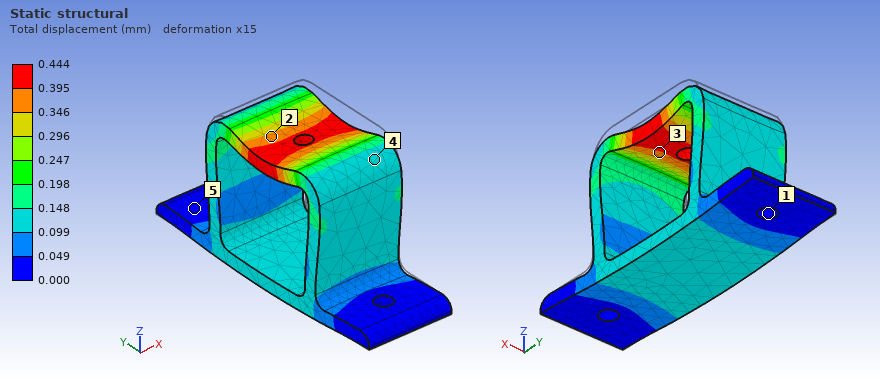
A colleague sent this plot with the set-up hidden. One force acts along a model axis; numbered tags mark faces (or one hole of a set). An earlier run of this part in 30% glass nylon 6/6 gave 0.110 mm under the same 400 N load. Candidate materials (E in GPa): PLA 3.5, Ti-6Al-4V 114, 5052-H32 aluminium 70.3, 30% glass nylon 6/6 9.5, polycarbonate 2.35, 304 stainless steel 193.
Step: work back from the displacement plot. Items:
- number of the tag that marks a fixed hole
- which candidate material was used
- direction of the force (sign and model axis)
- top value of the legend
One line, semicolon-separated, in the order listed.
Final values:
1; polycarbonate; -Z; 0.444 mm
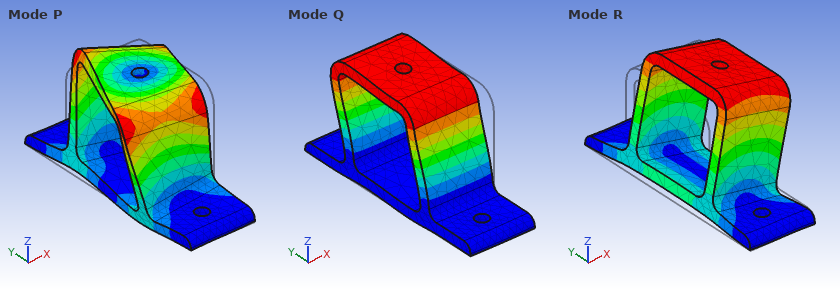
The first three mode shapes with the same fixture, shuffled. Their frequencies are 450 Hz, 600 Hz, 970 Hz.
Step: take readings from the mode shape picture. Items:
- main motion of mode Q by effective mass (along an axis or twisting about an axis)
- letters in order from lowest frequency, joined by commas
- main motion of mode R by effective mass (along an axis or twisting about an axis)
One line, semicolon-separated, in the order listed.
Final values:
along Y; R, Q, P; along X
